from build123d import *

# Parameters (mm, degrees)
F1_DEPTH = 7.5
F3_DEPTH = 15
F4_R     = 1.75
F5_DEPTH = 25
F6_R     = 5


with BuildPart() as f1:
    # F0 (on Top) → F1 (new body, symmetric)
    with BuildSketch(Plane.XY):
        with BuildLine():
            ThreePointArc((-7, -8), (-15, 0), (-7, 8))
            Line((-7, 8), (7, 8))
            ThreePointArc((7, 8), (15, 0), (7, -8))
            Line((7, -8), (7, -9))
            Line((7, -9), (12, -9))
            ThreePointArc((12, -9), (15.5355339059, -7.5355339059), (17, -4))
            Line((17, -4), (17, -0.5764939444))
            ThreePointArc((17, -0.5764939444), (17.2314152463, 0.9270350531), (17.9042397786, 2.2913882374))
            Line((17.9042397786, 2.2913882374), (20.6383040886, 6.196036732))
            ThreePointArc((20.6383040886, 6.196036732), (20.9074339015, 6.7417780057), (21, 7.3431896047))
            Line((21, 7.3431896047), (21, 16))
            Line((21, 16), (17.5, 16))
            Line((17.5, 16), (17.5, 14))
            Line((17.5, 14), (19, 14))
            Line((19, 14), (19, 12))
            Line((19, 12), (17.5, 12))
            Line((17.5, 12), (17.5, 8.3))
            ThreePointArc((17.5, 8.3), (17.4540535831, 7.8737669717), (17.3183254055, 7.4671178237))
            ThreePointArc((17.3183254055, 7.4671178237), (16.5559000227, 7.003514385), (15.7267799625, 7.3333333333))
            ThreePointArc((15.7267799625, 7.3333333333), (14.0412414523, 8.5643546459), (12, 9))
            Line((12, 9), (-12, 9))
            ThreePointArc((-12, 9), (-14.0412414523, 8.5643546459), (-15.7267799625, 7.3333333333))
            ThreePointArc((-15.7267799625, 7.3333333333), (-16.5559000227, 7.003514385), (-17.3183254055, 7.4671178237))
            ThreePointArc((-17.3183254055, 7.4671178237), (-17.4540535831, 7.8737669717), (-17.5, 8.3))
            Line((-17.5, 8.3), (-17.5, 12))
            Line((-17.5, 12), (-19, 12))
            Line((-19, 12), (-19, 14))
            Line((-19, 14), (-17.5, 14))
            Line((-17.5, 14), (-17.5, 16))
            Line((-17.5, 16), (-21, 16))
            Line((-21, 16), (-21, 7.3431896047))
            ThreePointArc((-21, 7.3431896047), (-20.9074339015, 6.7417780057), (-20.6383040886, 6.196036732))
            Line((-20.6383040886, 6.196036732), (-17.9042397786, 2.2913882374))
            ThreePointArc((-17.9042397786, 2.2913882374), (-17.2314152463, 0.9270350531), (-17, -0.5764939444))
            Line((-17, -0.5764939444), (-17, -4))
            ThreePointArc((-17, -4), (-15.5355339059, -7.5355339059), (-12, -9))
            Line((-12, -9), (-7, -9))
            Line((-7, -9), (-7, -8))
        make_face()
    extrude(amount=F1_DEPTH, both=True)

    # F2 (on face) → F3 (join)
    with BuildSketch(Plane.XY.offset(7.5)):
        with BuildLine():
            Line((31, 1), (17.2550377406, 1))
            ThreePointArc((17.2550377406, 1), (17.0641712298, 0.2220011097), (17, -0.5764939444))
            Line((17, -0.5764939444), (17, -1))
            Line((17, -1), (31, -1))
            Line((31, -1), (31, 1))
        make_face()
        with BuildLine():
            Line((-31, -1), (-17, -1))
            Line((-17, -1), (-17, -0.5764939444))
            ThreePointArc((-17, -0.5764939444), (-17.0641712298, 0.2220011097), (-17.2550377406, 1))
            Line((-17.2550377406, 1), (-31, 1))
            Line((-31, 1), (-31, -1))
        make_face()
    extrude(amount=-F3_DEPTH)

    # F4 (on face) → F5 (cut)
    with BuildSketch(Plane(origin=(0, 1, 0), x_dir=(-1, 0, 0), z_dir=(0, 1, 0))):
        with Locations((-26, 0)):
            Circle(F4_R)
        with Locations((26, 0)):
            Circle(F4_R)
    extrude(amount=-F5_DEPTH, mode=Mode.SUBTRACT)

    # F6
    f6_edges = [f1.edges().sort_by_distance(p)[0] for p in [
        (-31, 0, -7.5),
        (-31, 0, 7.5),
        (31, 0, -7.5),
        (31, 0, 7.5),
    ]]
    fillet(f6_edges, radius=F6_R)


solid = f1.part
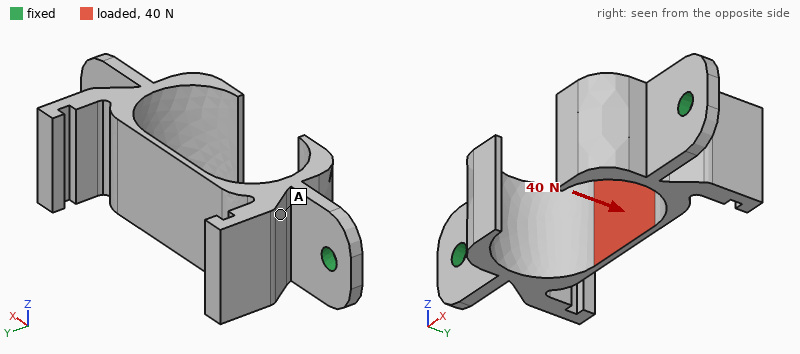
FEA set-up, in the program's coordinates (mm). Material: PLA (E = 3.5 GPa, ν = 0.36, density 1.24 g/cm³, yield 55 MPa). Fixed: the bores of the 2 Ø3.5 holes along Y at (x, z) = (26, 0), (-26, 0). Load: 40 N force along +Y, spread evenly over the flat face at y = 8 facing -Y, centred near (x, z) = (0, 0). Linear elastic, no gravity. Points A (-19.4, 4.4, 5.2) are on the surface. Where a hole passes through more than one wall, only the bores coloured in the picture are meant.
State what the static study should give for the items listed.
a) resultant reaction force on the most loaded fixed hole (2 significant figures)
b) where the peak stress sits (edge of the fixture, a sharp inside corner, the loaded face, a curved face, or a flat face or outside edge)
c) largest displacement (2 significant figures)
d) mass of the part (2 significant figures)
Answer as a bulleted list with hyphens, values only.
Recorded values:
- 41 N
- a flat face or outside edge
- 0.30 mm
- 5.3 g
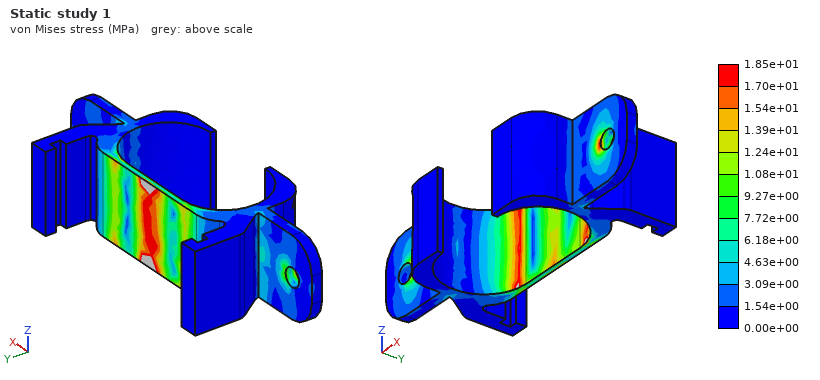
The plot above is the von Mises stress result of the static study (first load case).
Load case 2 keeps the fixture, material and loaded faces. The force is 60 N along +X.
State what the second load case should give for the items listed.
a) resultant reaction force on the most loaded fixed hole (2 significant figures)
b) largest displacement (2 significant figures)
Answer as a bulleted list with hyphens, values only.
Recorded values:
- 31 N
- 0.42 mm
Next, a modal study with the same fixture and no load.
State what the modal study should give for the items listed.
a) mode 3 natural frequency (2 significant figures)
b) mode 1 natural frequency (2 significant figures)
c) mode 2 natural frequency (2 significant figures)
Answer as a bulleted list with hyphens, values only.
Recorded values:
- 1500 Hz
- 1100 Hz
- 1100 Hz
